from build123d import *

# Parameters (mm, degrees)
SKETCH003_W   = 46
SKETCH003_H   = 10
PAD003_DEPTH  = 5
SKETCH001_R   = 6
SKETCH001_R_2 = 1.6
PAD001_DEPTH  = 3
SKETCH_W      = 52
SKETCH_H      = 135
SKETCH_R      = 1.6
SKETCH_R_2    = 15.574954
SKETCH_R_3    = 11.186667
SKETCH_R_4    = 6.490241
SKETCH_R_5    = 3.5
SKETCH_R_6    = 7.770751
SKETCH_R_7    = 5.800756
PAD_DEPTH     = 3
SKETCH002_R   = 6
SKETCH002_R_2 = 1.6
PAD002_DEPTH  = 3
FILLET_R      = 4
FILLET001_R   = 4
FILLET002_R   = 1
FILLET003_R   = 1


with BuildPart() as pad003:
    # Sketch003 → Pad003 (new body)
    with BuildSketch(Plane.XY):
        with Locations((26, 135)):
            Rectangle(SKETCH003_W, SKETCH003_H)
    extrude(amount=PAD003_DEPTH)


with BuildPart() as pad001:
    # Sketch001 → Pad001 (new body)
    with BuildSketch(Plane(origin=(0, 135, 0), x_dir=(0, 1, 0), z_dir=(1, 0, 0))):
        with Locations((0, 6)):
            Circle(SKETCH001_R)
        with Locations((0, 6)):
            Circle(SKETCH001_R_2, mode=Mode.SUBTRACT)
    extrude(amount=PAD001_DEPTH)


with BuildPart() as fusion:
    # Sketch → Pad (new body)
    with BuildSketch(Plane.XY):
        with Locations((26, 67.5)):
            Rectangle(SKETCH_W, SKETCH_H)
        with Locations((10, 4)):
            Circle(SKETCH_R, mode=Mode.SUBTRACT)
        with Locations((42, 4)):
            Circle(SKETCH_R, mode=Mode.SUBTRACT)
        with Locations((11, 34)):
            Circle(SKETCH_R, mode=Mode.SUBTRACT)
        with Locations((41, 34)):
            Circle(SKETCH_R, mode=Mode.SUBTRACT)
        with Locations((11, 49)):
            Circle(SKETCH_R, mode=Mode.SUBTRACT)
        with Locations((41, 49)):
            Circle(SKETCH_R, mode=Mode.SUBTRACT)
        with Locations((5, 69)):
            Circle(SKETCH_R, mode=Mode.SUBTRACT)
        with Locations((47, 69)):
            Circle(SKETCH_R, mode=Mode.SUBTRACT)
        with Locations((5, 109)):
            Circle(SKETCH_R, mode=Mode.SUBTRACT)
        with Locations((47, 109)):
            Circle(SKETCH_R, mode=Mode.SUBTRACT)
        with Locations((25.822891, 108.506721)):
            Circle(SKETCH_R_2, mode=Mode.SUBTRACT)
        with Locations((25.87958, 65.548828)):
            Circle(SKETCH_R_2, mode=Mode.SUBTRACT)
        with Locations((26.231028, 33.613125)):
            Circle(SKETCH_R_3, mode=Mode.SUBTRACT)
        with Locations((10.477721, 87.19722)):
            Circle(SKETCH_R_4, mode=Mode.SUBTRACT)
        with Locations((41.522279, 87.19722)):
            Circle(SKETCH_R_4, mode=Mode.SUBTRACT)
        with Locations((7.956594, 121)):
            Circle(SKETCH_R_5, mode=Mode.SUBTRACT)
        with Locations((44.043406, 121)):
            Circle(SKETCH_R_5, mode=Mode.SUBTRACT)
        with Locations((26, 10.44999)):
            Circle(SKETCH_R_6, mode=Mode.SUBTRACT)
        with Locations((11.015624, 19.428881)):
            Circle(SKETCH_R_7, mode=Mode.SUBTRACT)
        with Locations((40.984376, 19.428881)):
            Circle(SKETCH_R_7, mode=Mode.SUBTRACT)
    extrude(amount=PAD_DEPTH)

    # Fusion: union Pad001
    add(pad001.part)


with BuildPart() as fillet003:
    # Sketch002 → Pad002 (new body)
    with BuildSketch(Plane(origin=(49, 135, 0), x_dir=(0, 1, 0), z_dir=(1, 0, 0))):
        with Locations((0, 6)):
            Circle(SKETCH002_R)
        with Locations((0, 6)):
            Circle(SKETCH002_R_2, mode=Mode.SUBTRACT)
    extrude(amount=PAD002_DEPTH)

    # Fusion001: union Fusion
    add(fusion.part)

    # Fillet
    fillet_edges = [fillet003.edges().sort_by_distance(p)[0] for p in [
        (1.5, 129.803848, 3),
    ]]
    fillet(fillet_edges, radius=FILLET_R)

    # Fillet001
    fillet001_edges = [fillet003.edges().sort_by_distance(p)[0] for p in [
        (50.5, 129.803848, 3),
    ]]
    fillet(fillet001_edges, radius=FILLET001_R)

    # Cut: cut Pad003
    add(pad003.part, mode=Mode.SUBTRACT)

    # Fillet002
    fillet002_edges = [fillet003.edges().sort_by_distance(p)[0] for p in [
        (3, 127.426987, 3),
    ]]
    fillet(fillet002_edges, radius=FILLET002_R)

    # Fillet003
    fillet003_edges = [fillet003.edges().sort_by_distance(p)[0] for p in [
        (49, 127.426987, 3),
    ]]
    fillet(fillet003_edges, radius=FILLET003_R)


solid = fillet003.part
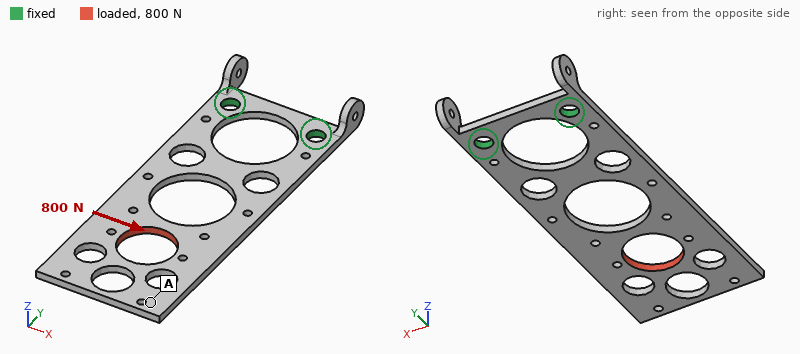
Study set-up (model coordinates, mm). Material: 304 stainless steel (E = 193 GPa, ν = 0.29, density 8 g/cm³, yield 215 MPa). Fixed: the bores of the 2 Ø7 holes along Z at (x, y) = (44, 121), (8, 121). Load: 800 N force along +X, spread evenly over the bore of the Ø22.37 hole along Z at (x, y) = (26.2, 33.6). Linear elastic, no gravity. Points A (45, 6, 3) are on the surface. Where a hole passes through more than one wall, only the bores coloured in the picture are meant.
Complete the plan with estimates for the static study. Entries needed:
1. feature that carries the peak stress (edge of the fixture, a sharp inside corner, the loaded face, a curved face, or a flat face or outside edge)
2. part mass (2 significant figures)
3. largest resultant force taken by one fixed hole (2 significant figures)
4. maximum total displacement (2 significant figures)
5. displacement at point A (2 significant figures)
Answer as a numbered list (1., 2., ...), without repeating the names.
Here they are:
1. a curved face
2. 100 g
3. 1.5 kN
4. 0.12 mm
5. 0.12 mm
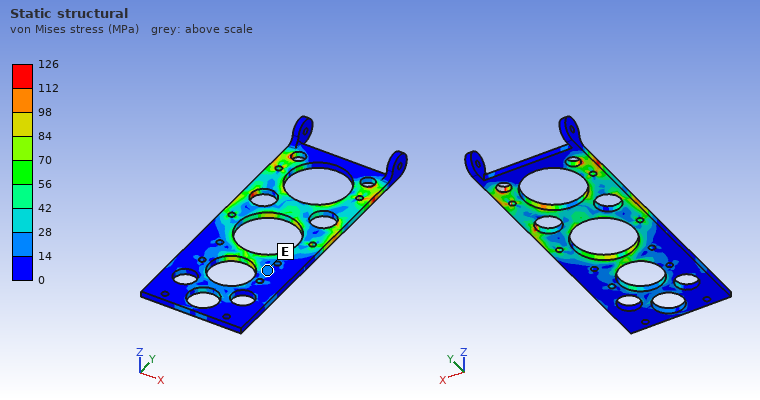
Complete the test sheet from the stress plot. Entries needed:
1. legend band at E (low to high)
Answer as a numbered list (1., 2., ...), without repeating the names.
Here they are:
1. 14 to 28 MPa
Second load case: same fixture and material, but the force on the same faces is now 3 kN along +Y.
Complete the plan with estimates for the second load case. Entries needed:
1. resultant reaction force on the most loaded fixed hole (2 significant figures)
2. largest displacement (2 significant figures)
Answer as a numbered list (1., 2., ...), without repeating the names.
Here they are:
1. 1.5 kN
2. 31 µm
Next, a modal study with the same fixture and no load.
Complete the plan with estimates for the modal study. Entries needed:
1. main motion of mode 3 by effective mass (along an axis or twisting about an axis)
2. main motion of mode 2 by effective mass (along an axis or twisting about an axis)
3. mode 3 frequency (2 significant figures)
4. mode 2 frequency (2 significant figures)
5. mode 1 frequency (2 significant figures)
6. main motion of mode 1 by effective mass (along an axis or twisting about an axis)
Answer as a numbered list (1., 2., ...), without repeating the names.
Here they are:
1. along Z
2. twisting about Y
3. 900 Hz
4. 610 Hz
5. 130 Hz
6. along Z
